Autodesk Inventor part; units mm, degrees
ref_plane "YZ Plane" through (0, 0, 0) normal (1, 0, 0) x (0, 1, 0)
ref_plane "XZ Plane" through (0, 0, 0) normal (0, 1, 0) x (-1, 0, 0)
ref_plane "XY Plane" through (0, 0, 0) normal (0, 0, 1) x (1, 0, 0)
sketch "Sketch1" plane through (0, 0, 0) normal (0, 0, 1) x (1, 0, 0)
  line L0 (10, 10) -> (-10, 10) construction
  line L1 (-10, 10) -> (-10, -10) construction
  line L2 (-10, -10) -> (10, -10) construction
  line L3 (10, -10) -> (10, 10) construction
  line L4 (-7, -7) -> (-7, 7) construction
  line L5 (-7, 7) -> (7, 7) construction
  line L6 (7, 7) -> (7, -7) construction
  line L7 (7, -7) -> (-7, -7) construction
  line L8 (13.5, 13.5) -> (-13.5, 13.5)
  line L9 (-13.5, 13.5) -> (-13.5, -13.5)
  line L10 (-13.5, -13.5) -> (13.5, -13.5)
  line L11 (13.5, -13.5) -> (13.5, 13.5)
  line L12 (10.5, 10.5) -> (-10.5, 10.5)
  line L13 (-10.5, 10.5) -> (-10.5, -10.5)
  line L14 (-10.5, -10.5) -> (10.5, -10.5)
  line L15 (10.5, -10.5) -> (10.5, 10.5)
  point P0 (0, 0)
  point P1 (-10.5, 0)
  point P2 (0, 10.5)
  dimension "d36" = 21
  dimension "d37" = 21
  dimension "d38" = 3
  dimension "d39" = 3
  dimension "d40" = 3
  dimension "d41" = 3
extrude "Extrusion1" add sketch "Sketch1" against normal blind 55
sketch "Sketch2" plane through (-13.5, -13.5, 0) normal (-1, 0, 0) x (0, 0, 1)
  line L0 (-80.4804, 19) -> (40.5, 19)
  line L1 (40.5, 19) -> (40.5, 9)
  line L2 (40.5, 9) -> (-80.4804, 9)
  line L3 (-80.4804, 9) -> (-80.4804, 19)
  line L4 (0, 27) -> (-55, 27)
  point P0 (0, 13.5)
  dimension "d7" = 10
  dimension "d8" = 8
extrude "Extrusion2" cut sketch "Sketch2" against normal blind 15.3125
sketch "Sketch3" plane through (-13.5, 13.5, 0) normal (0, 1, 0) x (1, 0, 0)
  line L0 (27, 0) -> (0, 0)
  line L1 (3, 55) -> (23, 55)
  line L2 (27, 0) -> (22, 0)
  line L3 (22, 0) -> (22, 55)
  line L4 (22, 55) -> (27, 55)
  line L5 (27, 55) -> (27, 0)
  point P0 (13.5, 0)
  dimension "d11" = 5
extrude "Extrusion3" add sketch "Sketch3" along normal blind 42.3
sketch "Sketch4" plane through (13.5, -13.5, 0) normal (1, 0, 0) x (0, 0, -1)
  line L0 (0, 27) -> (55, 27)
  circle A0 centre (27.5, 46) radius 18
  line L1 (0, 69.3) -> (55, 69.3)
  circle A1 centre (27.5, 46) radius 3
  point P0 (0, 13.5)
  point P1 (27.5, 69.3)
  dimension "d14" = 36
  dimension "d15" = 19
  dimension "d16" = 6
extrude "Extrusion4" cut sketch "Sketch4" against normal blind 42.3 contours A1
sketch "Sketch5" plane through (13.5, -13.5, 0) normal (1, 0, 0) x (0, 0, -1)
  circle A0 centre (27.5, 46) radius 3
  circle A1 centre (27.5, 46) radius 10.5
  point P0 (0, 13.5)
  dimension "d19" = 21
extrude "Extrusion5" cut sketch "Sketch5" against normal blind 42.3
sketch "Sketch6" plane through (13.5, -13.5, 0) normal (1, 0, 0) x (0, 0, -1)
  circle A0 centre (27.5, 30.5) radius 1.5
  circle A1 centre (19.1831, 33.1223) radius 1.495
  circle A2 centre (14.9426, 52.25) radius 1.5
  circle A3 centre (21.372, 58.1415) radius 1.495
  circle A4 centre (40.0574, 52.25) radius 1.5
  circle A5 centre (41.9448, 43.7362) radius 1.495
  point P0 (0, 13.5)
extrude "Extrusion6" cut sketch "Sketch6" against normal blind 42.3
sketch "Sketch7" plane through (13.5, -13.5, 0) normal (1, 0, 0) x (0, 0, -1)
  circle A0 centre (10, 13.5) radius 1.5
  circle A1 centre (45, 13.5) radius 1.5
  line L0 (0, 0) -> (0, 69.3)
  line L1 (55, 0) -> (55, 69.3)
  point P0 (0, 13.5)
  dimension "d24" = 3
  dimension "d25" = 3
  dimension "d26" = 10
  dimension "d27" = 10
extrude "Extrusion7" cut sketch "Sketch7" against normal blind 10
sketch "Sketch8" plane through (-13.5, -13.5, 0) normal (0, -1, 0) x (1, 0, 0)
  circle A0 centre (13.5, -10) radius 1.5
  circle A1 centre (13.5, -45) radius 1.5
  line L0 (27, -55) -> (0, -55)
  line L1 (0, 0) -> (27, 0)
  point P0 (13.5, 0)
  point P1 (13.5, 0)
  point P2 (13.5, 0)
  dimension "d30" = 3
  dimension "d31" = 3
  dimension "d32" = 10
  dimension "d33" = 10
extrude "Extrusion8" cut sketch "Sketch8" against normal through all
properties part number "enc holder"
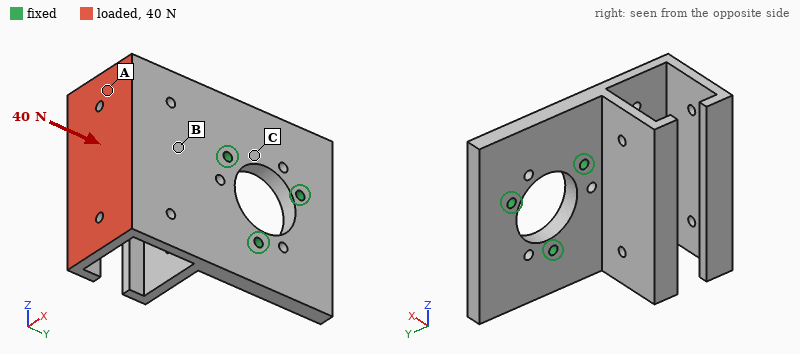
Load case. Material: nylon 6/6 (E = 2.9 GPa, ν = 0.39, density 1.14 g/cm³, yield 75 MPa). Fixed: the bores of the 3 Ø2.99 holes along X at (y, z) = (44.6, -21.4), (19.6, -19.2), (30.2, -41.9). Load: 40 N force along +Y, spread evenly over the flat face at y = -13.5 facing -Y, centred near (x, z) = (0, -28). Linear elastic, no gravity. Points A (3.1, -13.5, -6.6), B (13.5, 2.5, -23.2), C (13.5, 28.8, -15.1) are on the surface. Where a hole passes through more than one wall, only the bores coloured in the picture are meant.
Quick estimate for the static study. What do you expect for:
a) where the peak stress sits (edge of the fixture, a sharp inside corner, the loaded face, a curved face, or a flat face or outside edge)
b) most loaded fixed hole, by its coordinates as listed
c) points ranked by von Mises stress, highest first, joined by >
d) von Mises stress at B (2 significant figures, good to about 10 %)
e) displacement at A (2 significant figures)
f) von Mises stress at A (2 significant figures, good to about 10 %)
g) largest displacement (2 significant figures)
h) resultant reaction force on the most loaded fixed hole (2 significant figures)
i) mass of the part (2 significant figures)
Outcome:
a curved face
(19.6, -19.2)
B > A > C
5.1 MPa
0.57 mm
2.2 MPa
1.1 mm
22 N
27 g
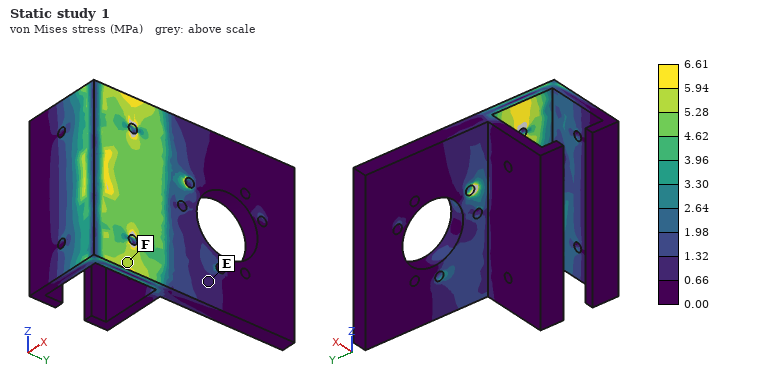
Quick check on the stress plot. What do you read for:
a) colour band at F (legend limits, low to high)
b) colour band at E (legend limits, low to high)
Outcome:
5.28 to 5.94 MPa
0.66 to 1.32 MPa
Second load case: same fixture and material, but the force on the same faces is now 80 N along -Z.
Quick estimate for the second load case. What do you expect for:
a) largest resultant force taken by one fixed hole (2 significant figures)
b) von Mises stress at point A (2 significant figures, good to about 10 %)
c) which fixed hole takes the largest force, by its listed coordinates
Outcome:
110 N
2.4 MPa
(19.6, -19.2)
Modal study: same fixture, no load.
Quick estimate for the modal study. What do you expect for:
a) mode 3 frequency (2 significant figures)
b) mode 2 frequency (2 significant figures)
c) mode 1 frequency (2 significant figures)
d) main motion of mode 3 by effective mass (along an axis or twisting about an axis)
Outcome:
750 Hz
510 Hz
330 Hz
along X
